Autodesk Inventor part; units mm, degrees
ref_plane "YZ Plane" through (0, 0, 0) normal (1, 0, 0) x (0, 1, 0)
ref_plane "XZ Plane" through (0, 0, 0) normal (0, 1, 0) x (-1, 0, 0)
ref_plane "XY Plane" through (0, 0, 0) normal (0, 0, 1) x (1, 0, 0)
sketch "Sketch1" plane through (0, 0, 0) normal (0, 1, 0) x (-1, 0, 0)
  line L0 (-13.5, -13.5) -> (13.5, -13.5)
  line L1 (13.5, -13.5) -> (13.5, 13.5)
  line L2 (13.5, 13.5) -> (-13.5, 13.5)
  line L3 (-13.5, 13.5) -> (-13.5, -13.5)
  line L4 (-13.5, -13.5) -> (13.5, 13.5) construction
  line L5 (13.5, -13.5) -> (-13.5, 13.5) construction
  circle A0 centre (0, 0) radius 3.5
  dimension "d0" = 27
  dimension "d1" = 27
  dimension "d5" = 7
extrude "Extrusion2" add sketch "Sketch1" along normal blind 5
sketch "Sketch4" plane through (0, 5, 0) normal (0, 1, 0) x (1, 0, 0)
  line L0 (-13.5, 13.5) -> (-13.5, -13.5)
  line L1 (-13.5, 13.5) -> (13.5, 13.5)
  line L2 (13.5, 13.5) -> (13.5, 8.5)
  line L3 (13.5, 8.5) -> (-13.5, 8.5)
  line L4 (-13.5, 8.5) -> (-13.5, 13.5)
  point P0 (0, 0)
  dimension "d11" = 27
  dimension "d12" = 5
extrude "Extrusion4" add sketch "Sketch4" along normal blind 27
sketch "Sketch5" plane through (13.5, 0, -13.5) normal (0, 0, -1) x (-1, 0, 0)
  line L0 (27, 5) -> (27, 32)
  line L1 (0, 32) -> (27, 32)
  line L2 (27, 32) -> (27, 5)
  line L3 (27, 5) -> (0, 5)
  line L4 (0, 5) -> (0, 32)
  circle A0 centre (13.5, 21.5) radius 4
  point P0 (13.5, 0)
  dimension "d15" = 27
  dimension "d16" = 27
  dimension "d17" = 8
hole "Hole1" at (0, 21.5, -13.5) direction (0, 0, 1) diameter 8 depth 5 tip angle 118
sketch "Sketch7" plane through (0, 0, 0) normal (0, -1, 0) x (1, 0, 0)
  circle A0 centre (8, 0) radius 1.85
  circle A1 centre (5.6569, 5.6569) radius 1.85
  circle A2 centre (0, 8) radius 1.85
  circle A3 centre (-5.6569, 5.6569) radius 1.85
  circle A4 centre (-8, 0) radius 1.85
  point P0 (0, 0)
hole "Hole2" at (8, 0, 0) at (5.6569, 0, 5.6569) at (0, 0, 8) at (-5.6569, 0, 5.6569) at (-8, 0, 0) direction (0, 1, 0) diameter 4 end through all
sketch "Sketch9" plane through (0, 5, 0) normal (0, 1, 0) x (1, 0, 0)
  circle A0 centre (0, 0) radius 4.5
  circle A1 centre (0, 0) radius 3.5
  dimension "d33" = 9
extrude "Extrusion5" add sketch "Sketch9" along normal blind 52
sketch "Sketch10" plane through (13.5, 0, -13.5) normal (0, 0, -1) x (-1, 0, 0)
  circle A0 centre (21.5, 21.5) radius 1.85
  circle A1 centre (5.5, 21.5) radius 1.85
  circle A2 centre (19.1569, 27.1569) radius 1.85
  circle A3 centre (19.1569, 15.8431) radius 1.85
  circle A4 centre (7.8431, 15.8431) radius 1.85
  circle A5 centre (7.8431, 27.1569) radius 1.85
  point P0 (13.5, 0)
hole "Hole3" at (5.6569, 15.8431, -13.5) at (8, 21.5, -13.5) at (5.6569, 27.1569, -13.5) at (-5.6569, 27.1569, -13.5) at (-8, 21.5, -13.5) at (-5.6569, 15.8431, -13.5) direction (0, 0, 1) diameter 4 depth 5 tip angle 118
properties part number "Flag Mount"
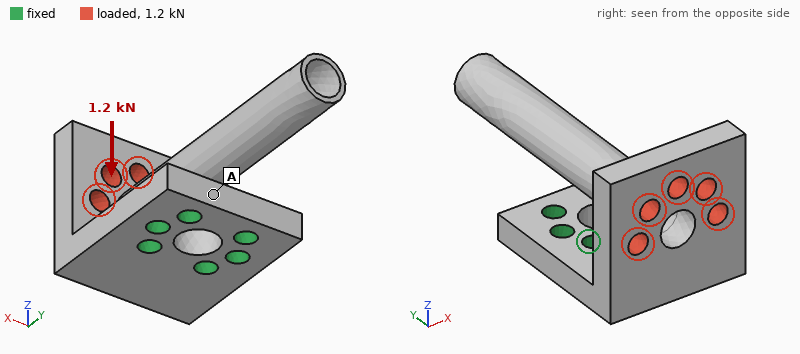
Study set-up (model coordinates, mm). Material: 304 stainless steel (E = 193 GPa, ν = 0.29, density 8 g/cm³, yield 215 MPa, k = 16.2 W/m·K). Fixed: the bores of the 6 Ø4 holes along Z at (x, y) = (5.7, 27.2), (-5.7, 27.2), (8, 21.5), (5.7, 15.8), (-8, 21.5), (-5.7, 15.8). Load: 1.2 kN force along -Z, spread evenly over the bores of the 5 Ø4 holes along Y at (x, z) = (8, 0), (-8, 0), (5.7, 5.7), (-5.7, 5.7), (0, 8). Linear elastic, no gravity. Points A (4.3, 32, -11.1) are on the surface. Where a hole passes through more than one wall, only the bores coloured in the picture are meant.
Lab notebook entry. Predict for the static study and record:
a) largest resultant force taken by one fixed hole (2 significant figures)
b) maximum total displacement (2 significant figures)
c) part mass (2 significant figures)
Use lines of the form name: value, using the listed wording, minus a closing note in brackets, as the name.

largest resultant force taken by one fixed hole: 780 N
maximum total displacement: 86 µm
part mass: 60 g
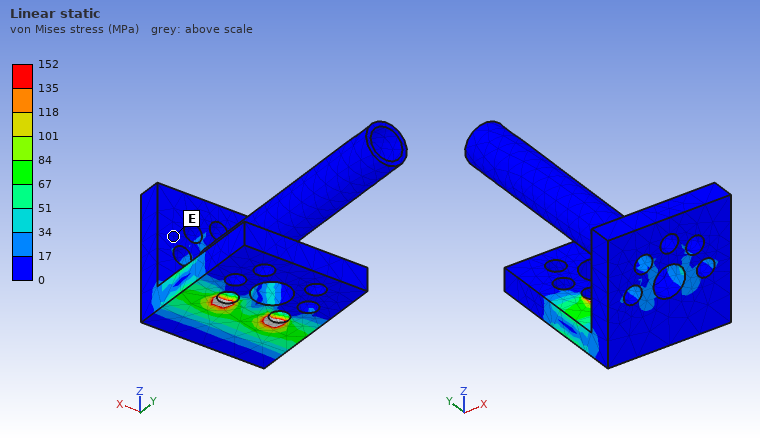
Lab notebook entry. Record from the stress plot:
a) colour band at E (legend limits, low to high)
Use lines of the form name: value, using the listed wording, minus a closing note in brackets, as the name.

colour band at E: 0 to 17 MPa
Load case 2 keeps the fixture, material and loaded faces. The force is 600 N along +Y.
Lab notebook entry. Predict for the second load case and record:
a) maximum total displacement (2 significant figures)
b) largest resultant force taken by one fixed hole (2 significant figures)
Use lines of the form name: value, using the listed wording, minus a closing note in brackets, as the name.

maximum total displacement: 0.16 mm
largest resultant force taken by one fixed hole: 300 N
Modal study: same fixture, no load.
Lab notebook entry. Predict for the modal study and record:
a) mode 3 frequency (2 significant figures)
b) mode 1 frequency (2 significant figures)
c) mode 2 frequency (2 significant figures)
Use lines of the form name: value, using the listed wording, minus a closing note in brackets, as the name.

mode 3 frequency: 4800 Hz
mode 1 frequency: 1700 Hz
mode 2 frequency: 2100 Hz
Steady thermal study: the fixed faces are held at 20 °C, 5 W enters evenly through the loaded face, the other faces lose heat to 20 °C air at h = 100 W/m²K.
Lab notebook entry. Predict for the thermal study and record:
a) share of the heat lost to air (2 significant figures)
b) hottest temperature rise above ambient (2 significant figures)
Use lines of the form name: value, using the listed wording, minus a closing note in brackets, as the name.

share of the heat lost to air: 75 %
hottest temperature rise above ambient: 26 K
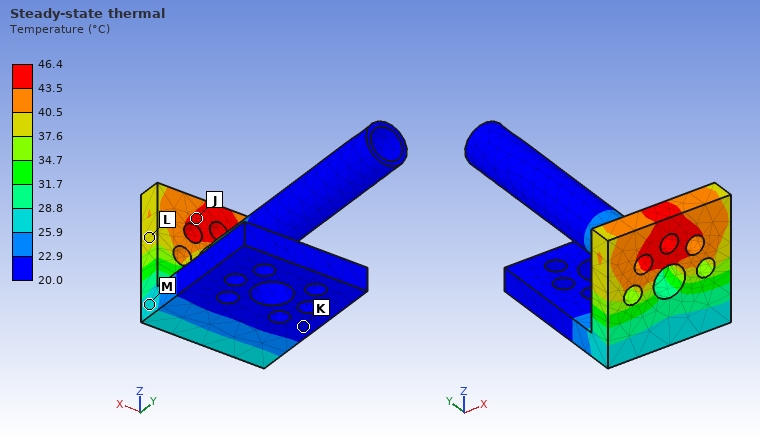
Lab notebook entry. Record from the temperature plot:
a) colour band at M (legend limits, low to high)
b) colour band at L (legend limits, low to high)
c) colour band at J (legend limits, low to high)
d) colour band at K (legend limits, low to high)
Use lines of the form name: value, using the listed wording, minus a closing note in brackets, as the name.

colour band at M: 25.9 to 28.8 °C
colour band at L: 37.6 to 40.5 °C
colour band at J: 43.5 to 46.4 °C
colour band at K: 20.0 to 22.9 °C
